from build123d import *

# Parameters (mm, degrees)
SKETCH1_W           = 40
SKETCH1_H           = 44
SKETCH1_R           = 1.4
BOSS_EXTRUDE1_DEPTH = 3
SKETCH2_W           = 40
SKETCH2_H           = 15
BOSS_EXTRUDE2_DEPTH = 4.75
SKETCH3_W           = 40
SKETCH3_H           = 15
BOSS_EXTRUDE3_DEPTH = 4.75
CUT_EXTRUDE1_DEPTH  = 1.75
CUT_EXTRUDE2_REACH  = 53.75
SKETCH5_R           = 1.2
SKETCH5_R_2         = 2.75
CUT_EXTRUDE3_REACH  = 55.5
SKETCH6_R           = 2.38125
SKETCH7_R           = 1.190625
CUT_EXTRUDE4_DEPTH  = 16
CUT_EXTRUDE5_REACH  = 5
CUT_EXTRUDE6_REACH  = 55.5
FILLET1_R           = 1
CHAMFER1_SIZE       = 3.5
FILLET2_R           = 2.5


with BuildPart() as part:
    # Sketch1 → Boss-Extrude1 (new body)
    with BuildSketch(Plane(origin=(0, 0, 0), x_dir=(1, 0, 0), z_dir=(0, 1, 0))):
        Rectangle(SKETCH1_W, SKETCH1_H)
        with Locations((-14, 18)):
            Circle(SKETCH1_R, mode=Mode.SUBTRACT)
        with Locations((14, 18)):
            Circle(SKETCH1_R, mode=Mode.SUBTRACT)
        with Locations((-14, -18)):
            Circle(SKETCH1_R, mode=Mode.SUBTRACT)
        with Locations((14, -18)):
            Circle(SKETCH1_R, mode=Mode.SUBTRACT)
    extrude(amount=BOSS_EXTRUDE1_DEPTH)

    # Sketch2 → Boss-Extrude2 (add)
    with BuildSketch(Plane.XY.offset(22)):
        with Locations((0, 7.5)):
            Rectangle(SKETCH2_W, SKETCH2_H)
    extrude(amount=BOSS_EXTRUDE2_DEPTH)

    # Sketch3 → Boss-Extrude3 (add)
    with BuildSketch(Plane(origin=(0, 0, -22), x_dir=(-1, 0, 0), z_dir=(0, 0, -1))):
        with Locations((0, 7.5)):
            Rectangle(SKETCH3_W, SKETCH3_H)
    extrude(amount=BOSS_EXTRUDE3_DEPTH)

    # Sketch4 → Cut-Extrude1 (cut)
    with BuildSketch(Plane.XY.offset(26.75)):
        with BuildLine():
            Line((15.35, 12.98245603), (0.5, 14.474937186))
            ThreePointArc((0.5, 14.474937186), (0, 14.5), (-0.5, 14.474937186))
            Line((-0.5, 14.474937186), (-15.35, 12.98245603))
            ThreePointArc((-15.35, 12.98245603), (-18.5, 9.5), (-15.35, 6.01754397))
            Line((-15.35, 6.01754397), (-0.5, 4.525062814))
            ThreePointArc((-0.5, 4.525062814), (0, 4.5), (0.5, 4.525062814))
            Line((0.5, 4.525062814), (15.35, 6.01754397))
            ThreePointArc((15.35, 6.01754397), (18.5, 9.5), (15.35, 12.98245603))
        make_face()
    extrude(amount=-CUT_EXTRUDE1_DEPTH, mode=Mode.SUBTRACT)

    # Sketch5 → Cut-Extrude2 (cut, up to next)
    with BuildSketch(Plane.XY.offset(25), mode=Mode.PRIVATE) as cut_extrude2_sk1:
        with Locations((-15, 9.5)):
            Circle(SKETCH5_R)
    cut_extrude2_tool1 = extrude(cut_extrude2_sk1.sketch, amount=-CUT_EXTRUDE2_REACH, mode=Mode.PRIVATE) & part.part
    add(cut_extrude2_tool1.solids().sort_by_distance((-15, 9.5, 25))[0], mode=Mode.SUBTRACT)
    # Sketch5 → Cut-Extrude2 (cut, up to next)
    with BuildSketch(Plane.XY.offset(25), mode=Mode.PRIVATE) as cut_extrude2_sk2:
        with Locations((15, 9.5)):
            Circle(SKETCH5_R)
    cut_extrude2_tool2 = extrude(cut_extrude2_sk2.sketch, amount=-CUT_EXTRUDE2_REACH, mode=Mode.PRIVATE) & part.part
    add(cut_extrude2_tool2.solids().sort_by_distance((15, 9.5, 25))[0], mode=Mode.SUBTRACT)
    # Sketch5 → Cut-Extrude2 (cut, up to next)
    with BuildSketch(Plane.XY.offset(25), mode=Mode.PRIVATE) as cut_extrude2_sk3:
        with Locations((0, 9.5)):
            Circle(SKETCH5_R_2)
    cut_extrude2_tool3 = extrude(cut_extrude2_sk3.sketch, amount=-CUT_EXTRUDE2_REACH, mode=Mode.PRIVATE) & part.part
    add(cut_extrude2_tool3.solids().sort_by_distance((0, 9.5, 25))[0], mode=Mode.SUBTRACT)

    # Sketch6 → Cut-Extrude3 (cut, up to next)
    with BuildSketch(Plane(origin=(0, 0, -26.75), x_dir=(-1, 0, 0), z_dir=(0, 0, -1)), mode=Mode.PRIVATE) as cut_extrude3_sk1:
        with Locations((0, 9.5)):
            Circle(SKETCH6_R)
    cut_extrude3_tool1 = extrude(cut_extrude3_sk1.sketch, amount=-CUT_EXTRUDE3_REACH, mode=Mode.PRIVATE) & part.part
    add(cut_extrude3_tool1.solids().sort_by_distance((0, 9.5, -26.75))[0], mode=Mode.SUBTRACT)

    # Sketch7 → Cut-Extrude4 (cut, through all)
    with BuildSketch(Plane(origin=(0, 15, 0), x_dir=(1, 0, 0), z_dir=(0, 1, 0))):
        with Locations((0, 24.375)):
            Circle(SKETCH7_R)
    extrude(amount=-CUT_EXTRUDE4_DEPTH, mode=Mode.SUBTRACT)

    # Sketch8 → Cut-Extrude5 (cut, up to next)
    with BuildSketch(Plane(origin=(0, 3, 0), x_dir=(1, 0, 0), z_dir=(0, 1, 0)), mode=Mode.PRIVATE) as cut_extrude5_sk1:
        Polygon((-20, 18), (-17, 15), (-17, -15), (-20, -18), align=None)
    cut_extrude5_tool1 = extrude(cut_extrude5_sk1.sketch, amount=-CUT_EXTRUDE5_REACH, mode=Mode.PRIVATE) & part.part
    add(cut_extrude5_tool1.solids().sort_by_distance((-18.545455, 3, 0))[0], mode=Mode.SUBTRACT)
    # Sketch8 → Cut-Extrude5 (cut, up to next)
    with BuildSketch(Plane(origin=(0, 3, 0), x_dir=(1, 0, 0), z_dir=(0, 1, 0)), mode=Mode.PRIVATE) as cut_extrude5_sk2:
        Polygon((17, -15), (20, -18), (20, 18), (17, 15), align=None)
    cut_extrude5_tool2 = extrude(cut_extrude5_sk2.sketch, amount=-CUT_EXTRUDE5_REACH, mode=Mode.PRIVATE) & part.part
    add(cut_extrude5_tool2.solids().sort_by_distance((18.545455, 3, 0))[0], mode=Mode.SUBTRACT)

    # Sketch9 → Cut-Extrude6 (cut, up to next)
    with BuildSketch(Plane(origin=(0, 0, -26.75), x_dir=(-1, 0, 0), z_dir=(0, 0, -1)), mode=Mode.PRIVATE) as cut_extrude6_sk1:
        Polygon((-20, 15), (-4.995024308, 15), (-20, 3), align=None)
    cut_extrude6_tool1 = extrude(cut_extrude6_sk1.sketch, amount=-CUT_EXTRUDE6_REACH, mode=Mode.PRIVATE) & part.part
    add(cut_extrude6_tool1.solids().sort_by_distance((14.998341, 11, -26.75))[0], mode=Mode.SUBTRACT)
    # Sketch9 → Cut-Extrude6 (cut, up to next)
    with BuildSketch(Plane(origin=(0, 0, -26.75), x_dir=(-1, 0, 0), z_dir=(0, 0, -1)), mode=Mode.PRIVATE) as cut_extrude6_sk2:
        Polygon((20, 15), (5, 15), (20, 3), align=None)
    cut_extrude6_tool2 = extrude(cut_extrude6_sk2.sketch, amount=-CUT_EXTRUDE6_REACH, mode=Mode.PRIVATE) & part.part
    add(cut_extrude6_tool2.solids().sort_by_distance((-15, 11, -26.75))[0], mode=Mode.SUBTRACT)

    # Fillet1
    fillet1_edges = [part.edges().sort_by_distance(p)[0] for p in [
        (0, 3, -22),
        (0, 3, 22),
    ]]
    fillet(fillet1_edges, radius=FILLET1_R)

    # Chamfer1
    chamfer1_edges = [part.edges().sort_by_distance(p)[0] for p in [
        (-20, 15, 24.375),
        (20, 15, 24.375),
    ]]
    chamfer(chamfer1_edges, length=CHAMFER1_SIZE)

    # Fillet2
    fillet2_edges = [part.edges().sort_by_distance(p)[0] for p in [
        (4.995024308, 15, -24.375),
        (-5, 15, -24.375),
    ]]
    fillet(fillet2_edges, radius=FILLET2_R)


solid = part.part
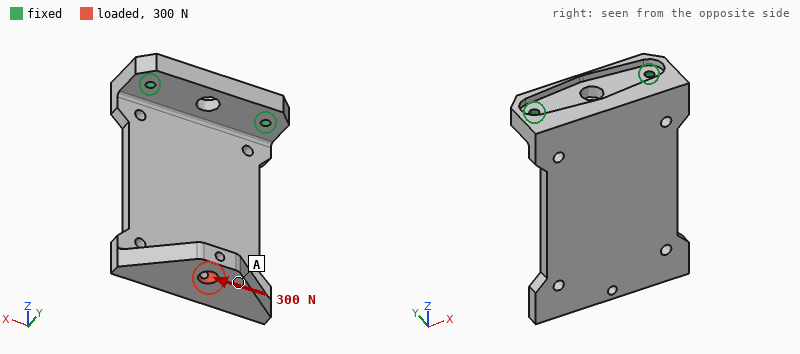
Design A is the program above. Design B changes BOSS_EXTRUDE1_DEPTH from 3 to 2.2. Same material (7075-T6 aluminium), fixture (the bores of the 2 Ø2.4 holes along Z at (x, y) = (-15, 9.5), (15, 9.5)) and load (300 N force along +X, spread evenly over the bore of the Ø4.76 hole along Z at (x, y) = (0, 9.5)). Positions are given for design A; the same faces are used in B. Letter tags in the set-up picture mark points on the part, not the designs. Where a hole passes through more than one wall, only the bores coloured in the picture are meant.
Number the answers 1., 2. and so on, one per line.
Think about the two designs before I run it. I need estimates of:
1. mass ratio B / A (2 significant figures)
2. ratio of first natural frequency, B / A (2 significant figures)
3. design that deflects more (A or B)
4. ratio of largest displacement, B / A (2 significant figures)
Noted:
1. 0.86
2. 0.74
3. B
4. 2.1
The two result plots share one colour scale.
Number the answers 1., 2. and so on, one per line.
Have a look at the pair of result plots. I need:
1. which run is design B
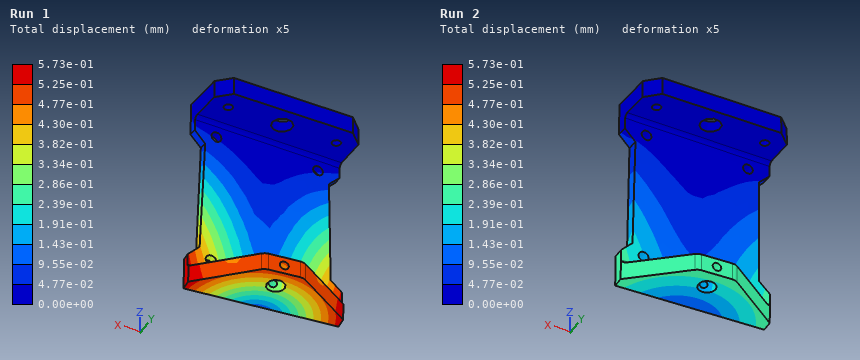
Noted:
1. Run 1
